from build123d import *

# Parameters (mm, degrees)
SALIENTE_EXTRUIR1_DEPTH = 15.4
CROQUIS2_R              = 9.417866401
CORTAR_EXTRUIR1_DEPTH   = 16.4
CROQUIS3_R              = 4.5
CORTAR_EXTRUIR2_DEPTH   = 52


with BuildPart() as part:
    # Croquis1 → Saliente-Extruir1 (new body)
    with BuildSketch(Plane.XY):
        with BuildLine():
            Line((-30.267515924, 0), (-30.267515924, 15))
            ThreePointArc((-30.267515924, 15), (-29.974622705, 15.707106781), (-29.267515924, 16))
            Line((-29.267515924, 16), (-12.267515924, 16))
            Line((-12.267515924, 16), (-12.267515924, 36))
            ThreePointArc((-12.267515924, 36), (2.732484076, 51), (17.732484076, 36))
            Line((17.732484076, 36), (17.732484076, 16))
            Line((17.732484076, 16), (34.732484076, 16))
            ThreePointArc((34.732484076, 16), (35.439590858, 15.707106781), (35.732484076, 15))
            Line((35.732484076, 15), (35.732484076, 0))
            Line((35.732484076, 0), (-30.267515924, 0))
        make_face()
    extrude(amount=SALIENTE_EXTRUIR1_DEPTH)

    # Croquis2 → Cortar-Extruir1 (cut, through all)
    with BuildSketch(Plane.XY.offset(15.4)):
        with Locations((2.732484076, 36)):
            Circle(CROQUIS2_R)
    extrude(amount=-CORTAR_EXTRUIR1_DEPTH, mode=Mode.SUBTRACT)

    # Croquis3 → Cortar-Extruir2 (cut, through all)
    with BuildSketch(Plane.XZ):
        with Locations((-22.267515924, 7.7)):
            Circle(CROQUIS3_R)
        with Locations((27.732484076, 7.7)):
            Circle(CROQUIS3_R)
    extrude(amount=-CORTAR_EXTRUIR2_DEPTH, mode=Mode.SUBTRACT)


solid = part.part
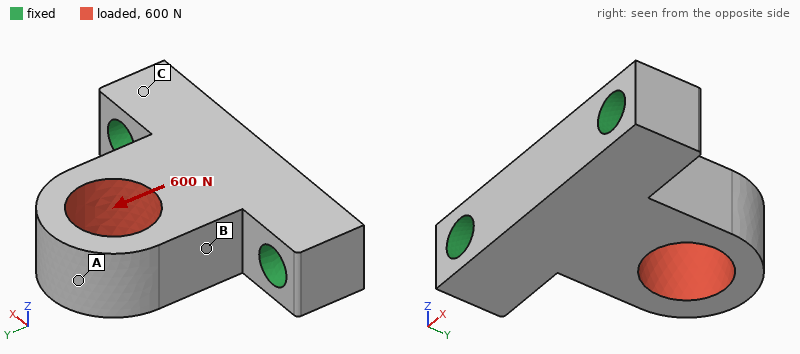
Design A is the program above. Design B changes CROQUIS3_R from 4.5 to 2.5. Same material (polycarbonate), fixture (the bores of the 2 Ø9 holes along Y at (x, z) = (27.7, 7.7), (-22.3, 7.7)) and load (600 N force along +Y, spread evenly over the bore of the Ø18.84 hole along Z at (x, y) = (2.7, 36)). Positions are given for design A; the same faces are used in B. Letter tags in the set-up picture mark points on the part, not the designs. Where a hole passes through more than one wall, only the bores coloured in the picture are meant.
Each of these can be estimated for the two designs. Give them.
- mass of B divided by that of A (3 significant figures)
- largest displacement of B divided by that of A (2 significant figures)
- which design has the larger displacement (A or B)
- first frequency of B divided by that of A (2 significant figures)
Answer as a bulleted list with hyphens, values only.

- 1.06
- 1.1
- B
- 0.92
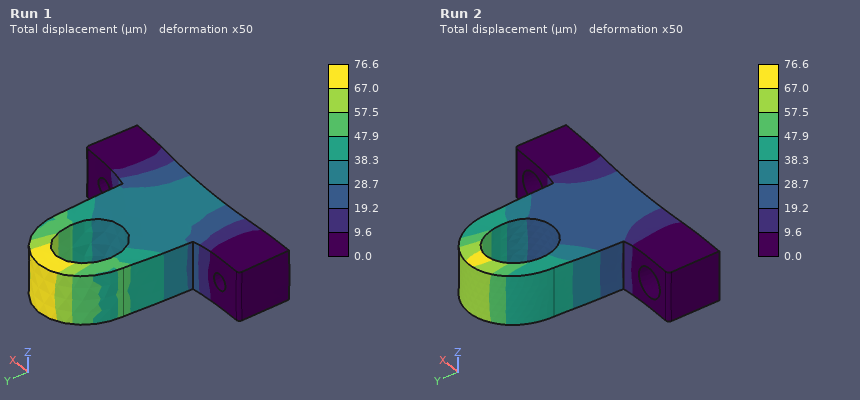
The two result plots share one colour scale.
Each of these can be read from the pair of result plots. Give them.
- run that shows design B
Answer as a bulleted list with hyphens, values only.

- Run 1
